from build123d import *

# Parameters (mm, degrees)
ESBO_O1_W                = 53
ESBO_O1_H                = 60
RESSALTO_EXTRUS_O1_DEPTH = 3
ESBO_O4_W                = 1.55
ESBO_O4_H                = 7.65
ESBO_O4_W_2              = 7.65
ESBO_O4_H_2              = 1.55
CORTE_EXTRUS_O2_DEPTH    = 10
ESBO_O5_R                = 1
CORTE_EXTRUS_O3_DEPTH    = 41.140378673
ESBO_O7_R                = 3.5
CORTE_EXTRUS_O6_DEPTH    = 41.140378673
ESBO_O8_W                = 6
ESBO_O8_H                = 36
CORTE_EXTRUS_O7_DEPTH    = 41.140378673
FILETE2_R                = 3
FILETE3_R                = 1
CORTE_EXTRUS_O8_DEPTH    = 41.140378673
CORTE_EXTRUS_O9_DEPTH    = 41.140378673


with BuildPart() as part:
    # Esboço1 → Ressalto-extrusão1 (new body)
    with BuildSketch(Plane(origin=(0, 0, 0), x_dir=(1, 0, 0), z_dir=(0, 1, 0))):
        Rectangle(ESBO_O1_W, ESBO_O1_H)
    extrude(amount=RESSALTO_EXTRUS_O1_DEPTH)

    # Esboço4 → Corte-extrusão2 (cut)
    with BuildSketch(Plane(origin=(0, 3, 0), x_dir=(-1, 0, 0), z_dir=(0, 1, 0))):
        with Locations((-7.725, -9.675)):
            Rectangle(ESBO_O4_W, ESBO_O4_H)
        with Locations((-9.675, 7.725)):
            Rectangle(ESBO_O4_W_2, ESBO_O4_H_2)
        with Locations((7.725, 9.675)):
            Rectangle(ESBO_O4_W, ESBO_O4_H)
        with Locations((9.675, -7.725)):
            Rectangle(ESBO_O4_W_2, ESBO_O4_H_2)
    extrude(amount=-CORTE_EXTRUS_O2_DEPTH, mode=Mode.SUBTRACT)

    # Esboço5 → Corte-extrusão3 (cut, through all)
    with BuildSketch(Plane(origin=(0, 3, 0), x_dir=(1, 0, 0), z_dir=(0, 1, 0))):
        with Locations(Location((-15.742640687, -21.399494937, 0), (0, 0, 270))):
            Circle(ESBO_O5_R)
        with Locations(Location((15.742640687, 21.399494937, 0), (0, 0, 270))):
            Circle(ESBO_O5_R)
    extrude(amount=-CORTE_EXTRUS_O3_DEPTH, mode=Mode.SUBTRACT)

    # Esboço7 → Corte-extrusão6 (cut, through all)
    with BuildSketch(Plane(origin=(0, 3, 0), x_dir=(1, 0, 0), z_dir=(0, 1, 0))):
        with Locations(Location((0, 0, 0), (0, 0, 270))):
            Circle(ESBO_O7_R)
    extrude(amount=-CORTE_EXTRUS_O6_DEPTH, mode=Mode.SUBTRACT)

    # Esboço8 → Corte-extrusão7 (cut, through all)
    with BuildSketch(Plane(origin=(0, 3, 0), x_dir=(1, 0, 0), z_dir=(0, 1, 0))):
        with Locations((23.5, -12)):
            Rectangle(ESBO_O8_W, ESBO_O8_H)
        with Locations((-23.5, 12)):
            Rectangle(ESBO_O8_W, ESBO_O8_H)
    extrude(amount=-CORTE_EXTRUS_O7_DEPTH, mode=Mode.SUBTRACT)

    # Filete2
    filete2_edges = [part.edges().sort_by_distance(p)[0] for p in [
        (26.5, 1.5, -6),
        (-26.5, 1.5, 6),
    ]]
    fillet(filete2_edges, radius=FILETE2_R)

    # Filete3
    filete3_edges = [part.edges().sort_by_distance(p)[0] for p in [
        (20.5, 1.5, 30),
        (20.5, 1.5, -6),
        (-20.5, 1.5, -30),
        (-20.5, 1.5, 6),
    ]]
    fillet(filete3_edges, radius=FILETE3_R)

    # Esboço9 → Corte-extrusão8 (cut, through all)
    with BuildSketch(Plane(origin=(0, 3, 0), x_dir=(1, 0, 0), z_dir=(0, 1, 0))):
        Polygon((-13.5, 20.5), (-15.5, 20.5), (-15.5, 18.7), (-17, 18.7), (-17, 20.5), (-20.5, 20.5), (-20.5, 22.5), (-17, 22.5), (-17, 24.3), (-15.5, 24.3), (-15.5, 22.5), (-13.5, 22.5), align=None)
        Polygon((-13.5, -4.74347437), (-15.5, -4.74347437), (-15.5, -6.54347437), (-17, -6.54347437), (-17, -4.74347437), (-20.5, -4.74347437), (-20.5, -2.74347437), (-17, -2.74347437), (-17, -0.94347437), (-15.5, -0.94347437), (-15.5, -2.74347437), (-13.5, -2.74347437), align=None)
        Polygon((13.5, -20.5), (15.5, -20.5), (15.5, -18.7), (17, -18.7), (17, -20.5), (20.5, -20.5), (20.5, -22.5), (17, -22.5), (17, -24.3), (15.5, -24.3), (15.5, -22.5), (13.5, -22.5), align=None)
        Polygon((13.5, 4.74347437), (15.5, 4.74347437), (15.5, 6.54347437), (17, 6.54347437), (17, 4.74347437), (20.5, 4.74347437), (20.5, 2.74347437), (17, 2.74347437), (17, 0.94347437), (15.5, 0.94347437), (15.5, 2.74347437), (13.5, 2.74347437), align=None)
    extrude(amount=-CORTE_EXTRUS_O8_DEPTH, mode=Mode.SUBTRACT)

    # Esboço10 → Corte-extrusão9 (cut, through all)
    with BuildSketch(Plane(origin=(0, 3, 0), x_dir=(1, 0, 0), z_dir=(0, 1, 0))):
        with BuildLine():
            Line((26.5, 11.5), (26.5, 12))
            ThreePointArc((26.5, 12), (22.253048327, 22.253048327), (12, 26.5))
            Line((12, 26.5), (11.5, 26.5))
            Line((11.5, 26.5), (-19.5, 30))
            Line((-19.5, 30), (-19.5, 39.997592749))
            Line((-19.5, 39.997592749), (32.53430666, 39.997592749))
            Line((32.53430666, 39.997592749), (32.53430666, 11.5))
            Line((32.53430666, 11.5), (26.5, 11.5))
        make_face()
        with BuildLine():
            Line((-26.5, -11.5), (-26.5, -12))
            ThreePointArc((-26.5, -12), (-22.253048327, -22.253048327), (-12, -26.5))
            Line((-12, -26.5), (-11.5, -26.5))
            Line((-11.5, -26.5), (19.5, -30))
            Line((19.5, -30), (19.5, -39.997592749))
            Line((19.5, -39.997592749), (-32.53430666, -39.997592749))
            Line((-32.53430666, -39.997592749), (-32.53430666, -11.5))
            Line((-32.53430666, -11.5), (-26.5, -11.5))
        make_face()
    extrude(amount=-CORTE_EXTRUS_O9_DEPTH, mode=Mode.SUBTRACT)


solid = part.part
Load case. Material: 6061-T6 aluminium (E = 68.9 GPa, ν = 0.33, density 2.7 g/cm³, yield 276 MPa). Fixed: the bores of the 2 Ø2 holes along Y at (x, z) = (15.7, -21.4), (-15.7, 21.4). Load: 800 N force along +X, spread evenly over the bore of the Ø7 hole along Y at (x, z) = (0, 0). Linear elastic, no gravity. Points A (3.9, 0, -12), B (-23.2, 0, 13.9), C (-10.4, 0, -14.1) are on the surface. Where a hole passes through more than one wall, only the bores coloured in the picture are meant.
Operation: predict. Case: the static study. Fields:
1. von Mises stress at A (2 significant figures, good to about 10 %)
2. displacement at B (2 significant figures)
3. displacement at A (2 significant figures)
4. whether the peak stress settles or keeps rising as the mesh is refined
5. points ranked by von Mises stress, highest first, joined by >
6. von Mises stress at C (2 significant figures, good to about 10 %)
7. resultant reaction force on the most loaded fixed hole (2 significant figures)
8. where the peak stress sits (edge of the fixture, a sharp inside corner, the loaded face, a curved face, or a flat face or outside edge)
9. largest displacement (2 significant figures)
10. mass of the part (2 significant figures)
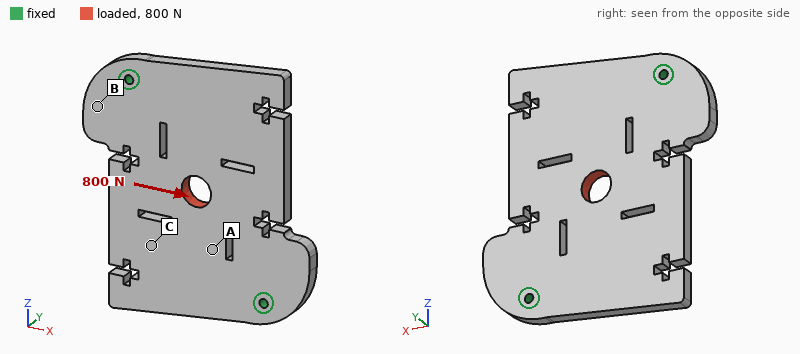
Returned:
13 MPa
5.5 µm
7.0 µm
keeps rising
A > C > B
7.2 MPa
400 N
edge of the fixture
14 µm
18 g
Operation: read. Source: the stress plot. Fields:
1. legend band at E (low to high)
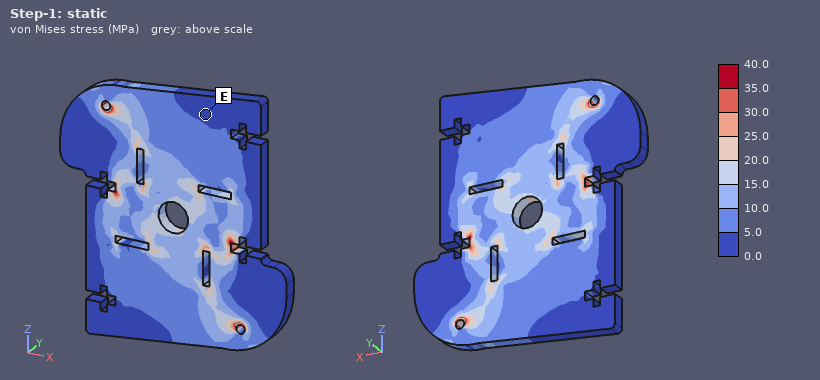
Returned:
0.0 to 5.0 MPa
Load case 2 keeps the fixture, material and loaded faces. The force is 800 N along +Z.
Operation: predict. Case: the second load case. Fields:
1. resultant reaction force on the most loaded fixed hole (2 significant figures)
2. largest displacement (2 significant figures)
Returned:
400 N
9.5 µm
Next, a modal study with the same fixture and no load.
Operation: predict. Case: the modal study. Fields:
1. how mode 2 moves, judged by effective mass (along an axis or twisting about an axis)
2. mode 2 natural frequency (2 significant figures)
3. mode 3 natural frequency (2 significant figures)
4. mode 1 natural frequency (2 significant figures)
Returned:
along Y
2600 Hz
5300 Hz
2000 Hz
